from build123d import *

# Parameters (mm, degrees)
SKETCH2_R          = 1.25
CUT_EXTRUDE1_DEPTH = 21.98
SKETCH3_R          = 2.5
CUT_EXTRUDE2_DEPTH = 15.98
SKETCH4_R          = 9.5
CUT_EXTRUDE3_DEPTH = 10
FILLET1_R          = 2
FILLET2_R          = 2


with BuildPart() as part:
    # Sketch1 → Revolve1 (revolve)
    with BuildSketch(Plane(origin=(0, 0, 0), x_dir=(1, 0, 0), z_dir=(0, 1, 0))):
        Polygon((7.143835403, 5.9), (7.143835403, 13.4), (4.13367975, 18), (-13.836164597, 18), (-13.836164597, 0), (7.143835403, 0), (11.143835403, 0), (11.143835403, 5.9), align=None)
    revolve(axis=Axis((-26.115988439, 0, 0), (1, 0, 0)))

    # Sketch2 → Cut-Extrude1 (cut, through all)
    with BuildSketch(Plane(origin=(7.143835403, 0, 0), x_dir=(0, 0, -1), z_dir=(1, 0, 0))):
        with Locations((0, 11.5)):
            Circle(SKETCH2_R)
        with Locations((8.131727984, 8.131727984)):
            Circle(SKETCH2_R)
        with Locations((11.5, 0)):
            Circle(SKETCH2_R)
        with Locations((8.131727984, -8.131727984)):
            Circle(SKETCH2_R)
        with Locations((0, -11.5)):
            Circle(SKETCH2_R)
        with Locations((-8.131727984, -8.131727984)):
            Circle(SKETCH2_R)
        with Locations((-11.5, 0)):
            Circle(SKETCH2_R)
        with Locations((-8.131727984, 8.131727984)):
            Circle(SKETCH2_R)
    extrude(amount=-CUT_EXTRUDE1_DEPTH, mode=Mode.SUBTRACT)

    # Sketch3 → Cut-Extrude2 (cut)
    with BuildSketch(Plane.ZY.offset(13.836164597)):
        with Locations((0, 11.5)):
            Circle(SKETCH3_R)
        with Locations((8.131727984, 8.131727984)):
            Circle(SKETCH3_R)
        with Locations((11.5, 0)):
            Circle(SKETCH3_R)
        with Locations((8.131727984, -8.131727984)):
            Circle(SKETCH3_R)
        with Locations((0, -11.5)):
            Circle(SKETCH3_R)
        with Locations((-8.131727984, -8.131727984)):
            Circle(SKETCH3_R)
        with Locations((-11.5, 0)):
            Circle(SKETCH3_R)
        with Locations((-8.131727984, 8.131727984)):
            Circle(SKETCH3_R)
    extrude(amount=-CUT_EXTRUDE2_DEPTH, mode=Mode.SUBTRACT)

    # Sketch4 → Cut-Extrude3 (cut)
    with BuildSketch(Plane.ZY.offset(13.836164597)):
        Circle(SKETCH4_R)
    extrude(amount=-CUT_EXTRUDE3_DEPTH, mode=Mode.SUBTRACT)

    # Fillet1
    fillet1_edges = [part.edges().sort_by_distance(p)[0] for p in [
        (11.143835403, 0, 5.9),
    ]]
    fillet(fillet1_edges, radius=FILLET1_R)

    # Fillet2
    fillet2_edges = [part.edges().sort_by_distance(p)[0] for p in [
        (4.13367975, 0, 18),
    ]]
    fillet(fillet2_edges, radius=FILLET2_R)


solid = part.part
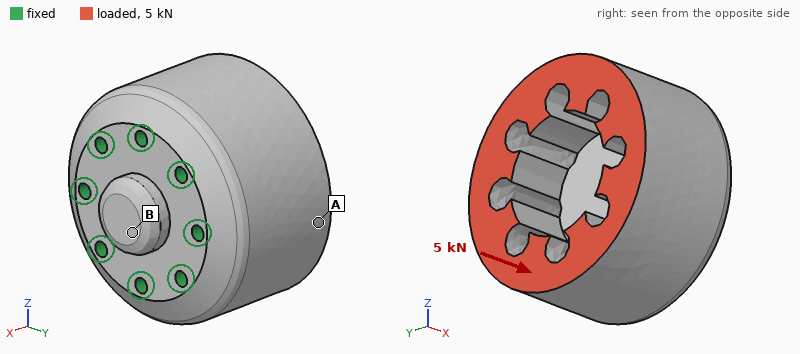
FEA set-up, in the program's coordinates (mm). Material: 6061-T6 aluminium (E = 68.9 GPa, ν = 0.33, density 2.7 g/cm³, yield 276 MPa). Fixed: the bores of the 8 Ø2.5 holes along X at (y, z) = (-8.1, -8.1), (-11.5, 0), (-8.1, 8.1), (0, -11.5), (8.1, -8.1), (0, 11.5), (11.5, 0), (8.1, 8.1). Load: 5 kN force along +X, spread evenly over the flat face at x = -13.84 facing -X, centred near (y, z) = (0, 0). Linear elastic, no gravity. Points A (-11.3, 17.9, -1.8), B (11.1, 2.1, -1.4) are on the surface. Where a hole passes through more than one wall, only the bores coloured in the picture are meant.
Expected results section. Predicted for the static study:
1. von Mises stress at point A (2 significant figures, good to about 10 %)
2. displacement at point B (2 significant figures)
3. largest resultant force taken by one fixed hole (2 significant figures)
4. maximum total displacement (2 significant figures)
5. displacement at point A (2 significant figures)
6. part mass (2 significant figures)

9.5 MPa
0.62 µm
630 N
4.1 µm
3.7 µm
42 g
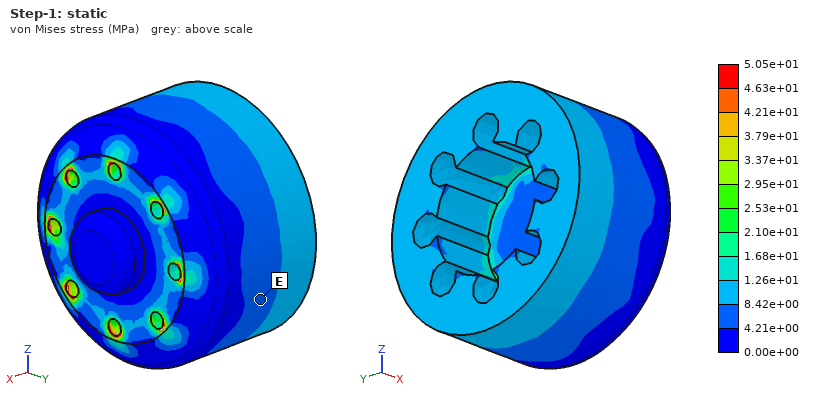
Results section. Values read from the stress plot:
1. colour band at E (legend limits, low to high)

4.21e+00 to 8.42e+00 MPa
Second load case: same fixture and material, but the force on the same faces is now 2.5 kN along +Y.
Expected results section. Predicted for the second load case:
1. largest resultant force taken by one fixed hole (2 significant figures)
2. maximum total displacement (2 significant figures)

850 N
15 µm
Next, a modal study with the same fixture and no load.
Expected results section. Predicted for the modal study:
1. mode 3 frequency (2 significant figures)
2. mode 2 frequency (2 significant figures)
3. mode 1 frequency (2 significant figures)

25 kHz
22 kHz
22 kHz
